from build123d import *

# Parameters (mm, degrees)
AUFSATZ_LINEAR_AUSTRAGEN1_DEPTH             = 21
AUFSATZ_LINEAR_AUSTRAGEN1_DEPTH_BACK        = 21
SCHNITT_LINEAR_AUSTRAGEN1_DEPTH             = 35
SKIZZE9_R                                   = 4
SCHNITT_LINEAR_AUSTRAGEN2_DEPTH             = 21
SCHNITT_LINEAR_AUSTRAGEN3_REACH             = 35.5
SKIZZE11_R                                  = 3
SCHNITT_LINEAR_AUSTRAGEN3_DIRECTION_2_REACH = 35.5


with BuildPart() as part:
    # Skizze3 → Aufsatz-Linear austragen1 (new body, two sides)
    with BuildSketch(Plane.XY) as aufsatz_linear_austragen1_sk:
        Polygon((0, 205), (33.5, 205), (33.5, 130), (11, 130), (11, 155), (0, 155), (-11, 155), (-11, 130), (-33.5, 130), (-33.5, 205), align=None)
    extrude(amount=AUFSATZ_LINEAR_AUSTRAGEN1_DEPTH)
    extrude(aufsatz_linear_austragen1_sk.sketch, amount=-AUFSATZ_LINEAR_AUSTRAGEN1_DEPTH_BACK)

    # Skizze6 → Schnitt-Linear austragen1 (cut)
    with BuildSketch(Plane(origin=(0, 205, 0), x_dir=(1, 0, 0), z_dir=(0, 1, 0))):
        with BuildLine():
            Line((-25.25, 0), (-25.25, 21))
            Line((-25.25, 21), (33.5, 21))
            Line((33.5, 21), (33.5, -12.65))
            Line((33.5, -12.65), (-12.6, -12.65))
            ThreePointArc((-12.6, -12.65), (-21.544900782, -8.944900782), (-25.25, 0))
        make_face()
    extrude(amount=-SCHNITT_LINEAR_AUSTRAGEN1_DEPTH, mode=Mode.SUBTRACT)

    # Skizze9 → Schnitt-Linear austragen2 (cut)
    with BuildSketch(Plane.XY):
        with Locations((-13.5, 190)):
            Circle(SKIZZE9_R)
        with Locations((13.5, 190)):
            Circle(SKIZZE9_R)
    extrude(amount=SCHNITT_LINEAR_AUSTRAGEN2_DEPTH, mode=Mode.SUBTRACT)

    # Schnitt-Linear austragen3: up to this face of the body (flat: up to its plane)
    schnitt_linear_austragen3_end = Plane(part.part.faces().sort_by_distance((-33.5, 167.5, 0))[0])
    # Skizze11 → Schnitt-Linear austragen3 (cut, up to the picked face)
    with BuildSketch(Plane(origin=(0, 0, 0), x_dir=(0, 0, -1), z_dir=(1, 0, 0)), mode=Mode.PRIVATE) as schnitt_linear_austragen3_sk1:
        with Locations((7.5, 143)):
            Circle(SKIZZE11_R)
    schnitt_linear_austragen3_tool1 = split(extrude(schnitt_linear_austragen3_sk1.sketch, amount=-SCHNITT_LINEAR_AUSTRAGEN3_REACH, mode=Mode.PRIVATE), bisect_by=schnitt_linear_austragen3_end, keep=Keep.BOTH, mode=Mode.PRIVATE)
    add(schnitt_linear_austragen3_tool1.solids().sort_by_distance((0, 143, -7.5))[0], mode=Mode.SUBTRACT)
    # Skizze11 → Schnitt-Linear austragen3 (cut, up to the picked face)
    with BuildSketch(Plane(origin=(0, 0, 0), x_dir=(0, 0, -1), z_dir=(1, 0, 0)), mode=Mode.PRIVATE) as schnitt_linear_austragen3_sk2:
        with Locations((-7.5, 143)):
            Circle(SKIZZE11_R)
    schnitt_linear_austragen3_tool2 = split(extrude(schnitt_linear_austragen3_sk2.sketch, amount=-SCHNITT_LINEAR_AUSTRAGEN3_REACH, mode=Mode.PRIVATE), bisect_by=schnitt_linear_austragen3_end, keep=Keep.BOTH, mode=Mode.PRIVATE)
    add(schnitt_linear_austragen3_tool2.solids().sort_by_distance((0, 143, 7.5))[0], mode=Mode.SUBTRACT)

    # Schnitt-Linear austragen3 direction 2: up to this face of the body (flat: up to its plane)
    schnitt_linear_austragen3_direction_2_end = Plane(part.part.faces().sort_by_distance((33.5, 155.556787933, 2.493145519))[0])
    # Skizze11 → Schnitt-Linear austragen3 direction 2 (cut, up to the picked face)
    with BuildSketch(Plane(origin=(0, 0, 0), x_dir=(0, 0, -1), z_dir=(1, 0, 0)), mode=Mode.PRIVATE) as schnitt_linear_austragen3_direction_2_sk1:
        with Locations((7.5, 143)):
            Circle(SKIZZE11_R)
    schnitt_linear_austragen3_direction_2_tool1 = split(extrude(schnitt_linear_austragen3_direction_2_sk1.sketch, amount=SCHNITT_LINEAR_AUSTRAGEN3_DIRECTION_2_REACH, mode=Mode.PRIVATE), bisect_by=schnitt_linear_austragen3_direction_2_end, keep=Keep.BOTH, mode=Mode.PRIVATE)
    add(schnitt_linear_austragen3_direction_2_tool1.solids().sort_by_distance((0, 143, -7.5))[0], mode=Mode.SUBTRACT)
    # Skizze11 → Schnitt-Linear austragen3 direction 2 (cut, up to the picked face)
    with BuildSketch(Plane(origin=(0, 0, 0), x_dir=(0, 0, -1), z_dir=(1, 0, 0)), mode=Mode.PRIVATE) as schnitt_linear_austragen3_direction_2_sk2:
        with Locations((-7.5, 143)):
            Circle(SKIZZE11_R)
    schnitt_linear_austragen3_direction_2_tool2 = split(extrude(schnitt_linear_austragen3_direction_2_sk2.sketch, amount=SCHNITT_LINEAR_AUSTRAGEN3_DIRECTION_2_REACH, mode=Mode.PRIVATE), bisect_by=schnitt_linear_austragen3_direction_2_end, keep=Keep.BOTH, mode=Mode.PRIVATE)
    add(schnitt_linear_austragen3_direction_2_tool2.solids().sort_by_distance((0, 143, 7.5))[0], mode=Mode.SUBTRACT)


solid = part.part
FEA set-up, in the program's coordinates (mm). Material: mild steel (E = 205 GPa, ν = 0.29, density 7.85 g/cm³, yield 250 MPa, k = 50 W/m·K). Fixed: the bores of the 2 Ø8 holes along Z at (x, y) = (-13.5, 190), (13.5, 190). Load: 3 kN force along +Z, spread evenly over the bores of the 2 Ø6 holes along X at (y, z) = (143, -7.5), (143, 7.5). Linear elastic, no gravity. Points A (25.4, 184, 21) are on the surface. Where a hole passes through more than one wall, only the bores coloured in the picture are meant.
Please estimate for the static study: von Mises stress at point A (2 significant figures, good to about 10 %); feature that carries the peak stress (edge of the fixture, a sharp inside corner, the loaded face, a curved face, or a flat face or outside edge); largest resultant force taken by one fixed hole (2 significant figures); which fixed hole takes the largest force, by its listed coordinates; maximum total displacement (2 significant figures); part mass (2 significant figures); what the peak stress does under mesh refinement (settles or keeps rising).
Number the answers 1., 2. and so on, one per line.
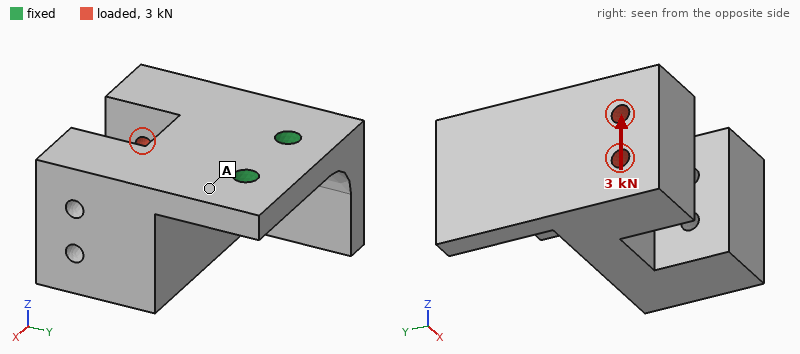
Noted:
1. 41 MPa
2. edge of the fixture
3. 3.1 kN
4. (-13.5, 190)
5. 0.13 mm
6. 920 g
7. keeps rising
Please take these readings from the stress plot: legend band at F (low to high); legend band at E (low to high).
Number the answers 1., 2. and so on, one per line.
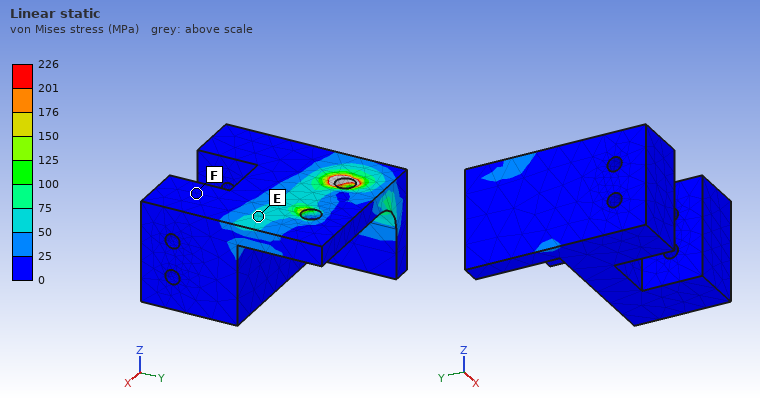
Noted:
1. 0 to 25 MPa
2. 50 to 75 MPa
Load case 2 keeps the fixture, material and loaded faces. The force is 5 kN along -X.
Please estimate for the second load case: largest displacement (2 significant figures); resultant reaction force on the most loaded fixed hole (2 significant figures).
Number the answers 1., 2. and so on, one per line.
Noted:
1. 48 µm
2. 7.7 kN
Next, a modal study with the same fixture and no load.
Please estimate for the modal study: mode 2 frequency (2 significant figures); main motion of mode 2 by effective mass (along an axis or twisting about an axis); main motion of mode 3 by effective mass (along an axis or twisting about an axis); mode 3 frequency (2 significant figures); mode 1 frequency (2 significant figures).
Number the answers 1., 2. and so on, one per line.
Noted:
1. 2500 Hz
2. along X
3. along X
4. 3800 Hz
5. 1300 Hz
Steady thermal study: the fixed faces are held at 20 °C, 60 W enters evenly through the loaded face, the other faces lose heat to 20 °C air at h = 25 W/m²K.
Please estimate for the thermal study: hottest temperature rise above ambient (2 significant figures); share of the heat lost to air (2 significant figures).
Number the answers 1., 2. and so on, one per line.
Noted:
1. 70 K
2. 30 %
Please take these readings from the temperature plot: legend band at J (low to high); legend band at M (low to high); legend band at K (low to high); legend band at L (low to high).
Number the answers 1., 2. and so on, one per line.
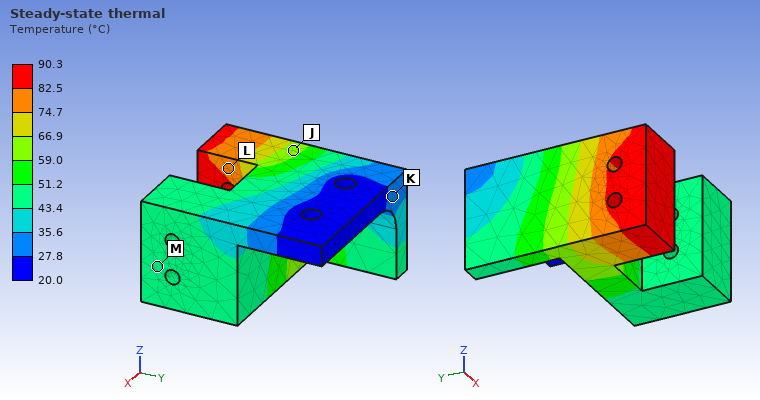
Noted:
1. 59.0 to 66.9 °C
2. 43.4 to 51.2 °C
3. 27.8 to 35.6 °C
4. 74.7 to 82.5 °C
